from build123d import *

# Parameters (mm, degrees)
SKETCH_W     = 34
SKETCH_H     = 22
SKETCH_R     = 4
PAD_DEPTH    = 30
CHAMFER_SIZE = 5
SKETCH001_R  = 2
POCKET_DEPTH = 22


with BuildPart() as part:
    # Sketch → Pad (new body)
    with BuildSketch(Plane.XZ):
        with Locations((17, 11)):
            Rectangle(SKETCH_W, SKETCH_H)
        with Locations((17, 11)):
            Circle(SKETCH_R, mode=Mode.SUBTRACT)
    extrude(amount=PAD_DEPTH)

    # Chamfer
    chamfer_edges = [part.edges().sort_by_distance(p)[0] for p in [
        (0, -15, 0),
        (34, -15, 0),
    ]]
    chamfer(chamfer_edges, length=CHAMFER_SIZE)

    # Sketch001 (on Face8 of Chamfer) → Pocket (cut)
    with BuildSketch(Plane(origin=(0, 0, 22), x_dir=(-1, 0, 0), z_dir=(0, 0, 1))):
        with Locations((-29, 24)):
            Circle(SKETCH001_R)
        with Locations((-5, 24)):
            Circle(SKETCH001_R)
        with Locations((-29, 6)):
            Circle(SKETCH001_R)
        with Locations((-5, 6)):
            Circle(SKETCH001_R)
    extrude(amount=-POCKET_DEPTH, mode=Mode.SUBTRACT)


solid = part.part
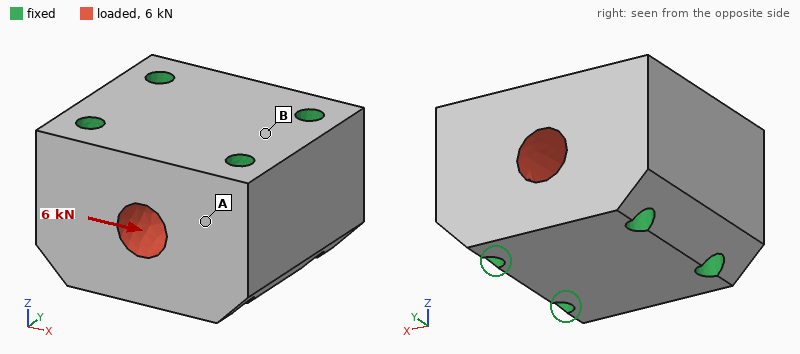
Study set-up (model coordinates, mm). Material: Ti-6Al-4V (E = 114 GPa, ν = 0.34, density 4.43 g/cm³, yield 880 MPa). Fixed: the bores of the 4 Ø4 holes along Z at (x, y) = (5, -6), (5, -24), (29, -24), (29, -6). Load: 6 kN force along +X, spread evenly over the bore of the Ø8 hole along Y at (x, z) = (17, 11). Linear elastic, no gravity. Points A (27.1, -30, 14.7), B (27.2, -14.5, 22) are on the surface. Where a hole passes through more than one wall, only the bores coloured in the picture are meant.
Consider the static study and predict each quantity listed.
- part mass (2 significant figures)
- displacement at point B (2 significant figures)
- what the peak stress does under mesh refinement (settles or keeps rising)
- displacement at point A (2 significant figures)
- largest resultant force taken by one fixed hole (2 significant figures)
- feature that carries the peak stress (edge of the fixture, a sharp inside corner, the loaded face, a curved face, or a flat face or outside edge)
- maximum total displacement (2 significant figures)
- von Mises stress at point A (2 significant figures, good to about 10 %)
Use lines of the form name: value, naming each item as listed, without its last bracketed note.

part mass: 85 g
displacement at point B: 0.33 µm
what the peak stress does under mesh refinement: keeps rising
displacement at point A: 0.27 µm
largest resultant force taken by one fixed hole: 1.5 kN
feature that carries the peak stress: edge of the fixture
maximum total displacement: 0.74 µm
von Mises stress at point A: 3.7 MPa
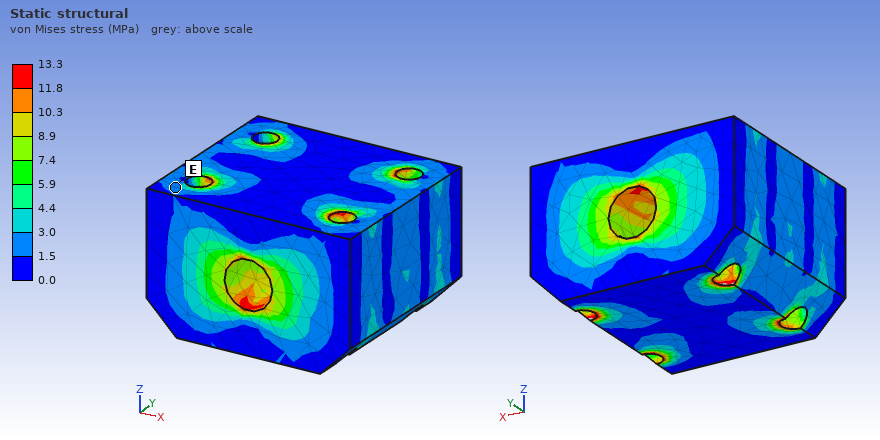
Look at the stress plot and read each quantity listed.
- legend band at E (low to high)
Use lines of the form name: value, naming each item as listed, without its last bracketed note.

legend band at E: 1.5 to 3.0 MPa
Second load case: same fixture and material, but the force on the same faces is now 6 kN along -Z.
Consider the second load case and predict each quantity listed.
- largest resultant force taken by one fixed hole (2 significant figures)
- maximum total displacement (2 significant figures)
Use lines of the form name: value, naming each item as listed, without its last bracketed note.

largest resultant force taken by one fixed hole: 1.5 kN
maximum total displacement: 1.6 µm
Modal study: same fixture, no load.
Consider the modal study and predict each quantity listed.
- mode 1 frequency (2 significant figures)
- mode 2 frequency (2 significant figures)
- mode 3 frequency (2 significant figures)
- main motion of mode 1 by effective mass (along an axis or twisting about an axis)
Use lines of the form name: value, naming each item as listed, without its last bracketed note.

mode 1 frequency: 60 kHz
mode 2 frequency: 63 kHz
mode 3 frequency: 66 kHz
main motion of mode 1 by effective mass: along Z
